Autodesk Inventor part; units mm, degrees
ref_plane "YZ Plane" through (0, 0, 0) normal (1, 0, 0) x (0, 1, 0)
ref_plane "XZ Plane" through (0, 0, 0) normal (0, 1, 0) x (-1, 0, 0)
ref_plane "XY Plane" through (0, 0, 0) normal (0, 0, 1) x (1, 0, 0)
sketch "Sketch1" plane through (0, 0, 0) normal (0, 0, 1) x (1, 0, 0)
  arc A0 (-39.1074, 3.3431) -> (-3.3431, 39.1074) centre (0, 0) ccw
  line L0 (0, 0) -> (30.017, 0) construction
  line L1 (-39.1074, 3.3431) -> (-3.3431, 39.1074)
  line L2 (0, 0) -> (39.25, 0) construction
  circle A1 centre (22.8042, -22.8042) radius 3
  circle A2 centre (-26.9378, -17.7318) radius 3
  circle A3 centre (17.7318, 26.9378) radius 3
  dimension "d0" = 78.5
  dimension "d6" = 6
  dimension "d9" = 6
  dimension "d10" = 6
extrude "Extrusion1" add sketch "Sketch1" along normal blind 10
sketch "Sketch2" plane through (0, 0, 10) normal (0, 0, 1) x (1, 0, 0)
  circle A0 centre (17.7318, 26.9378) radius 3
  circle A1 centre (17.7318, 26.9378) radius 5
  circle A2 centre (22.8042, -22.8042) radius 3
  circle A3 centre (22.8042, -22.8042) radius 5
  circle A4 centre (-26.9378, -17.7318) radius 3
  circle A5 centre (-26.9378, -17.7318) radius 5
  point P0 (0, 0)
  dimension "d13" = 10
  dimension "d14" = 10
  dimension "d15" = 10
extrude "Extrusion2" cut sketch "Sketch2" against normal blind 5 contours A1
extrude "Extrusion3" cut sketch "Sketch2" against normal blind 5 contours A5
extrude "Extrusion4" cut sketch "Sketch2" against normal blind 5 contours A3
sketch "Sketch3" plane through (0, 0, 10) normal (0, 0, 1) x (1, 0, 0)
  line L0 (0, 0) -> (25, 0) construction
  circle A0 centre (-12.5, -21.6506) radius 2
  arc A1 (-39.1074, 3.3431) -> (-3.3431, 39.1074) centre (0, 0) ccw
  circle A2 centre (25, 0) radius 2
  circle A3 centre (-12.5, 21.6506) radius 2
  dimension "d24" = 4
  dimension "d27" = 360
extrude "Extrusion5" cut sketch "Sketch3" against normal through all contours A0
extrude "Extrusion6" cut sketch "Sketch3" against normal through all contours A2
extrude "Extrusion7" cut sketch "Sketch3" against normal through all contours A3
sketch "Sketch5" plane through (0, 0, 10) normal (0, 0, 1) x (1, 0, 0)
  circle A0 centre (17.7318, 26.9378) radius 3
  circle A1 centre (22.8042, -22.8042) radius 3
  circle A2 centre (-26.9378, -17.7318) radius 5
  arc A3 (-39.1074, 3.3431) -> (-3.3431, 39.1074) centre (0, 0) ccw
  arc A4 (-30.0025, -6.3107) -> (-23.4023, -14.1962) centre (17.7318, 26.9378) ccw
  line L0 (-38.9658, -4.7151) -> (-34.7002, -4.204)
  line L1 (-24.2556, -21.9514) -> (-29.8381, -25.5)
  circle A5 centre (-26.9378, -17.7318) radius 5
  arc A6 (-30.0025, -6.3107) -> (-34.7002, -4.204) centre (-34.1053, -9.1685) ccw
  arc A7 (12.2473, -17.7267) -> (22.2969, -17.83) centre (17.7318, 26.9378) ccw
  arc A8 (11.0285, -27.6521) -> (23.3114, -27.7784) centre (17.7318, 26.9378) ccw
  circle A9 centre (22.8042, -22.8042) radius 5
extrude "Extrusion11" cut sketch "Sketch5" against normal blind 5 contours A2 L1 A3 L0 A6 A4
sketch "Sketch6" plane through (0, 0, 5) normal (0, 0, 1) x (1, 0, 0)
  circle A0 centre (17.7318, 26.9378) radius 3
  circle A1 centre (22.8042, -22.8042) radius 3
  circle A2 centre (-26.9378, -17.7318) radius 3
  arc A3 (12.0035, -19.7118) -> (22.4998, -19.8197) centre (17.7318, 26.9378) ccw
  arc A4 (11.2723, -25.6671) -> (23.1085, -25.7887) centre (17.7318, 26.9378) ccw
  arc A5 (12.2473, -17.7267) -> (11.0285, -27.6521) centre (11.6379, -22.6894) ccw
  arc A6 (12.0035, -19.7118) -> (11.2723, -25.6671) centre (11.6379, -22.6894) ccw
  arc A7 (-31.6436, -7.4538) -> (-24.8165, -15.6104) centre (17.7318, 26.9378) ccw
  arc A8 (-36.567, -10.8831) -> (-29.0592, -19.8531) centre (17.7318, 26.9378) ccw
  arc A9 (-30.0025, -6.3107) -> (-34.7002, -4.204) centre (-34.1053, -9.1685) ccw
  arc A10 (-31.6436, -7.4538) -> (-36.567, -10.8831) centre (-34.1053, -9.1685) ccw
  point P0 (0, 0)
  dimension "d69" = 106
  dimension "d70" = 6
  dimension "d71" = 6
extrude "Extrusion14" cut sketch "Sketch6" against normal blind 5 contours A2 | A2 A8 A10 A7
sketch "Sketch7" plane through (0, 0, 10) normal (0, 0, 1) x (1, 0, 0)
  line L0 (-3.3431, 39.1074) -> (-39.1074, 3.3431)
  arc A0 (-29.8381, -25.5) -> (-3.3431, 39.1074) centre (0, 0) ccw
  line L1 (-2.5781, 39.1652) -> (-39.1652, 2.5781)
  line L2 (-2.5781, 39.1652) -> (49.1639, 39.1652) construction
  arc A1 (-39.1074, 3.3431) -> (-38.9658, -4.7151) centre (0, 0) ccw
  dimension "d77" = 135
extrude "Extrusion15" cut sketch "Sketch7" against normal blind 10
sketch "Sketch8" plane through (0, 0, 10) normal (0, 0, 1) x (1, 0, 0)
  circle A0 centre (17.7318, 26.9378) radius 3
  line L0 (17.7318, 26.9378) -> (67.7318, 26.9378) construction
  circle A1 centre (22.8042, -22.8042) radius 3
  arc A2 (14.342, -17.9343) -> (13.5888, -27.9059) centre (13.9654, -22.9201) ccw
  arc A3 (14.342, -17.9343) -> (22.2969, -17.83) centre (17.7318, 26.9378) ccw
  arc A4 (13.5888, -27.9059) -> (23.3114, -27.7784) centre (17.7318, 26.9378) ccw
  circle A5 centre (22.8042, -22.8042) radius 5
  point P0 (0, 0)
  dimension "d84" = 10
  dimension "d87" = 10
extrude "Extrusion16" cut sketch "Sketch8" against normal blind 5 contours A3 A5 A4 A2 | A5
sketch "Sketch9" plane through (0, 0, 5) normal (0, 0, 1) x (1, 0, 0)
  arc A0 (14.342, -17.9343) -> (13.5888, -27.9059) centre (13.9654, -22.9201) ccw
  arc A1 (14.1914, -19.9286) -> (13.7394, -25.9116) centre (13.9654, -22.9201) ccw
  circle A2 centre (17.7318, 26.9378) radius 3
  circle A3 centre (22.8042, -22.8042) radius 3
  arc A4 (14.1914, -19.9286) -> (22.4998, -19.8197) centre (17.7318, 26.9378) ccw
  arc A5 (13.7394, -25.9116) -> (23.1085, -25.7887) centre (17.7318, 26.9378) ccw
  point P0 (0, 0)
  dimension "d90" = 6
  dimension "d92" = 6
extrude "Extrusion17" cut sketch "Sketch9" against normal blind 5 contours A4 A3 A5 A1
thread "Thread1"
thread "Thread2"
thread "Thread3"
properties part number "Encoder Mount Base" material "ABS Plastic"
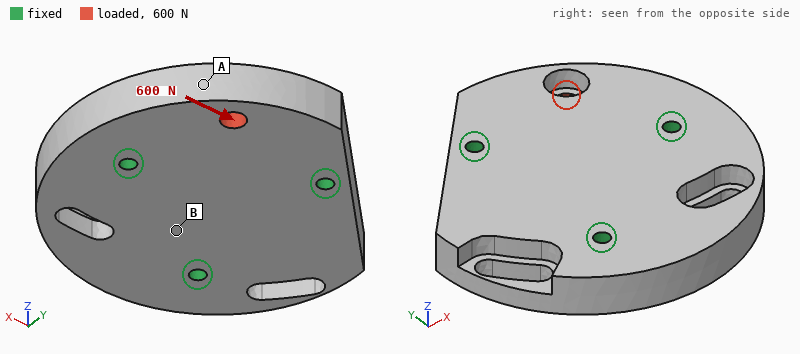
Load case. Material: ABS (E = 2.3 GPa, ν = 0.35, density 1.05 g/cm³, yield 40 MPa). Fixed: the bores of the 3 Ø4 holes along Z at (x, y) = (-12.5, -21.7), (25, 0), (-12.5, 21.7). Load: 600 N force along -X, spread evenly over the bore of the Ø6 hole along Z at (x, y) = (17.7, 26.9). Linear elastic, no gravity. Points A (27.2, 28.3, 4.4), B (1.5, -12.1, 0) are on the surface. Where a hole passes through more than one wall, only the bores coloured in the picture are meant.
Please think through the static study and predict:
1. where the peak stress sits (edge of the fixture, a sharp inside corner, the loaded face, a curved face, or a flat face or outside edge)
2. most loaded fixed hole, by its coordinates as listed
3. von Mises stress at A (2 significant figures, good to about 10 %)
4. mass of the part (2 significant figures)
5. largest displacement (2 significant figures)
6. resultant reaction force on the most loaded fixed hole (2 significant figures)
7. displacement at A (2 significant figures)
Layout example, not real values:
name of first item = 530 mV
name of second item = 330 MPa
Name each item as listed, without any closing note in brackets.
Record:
where the peak stress sits = the loaded face
most loaded fixed hole, by its coordinates as listed = (-12.5, 21.7)
von Mises stress at A = 2.0 MPa
mass of the part = 43 g
largest displacement = 81 µm
resultant reaction force on the most loaded fixed hole = 430 N
displacement at A = 67 µm
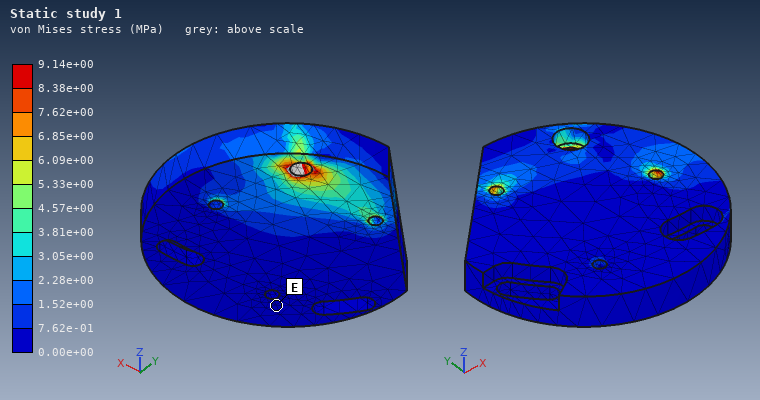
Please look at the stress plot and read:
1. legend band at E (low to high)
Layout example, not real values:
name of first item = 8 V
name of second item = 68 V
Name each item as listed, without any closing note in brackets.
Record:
legend band at E = 0.00e+00 to 7.62e-01 MPa
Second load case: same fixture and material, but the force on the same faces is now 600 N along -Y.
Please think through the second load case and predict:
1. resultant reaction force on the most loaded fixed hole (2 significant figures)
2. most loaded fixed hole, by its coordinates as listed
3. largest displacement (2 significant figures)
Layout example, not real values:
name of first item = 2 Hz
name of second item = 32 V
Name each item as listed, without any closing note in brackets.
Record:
resultant reaction force on the most loaded fixed hole = 430 N
most loaded fixed hole, by its coordinates as listed = (25, 0)
largest displacement = 0.10 mm
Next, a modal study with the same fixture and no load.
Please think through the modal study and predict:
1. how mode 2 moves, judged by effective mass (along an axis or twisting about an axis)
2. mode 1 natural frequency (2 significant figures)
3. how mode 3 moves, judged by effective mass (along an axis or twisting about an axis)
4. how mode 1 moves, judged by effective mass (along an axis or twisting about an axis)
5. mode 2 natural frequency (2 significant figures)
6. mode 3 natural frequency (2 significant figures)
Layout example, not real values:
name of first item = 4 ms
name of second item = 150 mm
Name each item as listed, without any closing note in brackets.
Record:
how mode 2 moves, judged by effective mass = twisting about Y
mode 1 natural frequency = 2800 Hz
how mode 3 moves, judged by effective mass = along Z
how mode 1 moves, judged by effective mass = twisting about X
mode 2 natural frequency = 2900 Hz
mode 3 natural frequency = 3500 Hz
